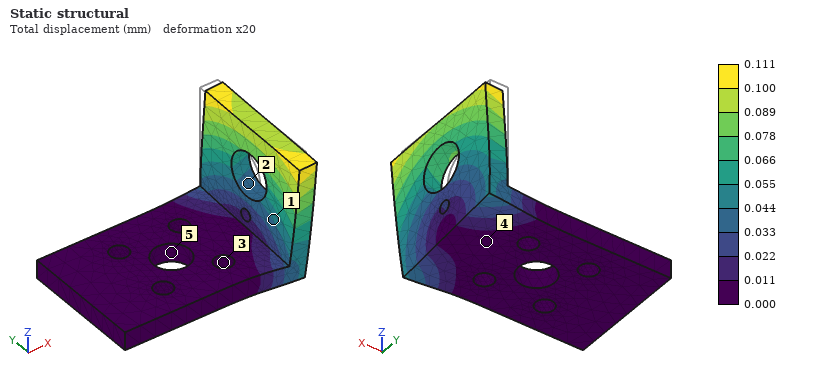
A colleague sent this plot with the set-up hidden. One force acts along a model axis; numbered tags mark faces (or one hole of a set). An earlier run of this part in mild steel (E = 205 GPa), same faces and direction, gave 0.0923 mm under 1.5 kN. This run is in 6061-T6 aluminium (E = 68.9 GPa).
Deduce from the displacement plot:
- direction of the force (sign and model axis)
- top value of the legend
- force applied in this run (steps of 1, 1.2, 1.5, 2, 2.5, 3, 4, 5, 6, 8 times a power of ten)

-Y
0.111 mm
600 N
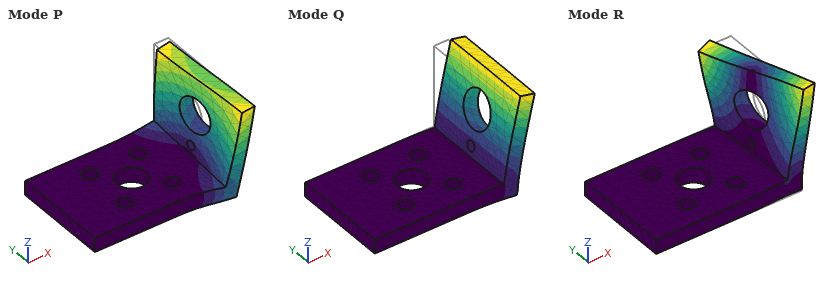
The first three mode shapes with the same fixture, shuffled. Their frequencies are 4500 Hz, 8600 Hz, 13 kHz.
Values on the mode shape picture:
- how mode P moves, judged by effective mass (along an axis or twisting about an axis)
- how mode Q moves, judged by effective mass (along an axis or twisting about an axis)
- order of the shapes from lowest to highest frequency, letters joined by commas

along Y
along X
Q, P, R
